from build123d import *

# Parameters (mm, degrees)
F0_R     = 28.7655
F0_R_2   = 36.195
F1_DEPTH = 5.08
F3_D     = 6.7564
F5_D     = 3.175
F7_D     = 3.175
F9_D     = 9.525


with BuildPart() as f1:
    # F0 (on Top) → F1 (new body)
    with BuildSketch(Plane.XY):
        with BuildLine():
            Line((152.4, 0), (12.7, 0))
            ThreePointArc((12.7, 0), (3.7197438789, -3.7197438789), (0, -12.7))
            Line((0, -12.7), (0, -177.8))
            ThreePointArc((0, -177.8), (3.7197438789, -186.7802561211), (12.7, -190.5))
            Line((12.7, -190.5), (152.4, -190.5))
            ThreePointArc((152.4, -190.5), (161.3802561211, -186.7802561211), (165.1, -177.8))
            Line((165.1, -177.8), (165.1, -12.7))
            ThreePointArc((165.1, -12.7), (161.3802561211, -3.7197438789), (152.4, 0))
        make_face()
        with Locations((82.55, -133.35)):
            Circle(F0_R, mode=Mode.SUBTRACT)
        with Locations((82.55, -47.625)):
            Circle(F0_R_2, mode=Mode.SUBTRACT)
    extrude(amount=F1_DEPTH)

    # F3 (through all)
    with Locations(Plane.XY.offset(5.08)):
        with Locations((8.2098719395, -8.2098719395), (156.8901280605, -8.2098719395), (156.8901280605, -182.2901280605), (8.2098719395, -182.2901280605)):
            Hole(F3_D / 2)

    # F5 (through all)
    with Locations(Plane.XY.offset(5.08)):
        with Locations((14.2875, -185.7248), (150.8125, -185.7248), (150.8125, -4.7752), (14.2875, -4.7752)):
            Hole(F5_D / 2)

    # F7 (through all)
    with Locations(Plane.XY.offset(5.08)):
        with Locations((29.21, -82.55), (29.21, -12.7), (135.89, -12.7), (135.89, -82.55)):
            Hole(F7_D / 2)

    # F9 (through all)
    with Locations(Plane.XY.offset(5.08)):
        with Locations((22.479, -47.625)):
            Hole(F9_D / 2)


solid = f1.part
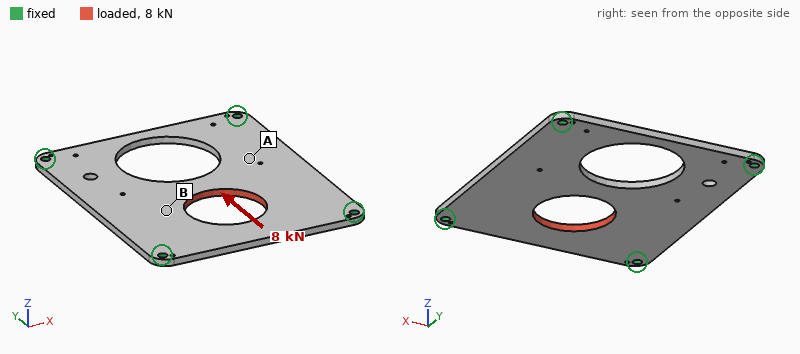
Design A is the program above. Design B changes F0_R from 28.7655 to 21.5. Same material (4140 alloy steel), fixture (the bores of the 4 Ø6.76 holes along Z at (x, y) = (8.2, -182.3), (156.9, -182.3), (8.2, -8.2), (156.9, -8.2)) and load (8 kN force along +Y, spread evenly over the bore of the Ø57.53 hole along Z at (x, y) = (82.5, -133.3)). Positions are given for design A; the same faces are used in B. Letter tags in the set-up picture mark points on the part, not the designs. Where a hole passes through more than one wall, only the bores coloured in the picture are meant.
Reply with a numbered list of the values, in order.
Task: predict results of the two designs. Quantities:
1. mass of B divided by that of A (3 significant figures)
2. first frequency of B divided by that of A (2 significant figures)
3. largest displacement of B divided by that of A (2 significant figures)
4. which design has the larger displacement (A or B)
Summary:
1. 1.05
2. 0.98
3. 0.90
4. A
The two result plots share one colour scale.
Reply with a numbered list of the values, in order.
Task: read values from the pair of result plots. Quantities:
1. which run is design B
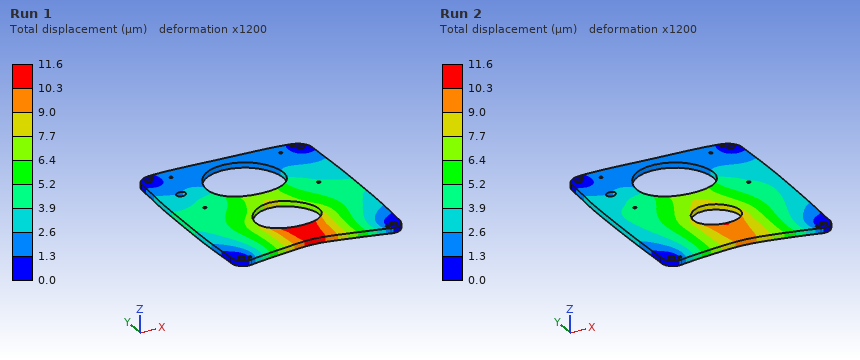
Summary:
1. Run 2
